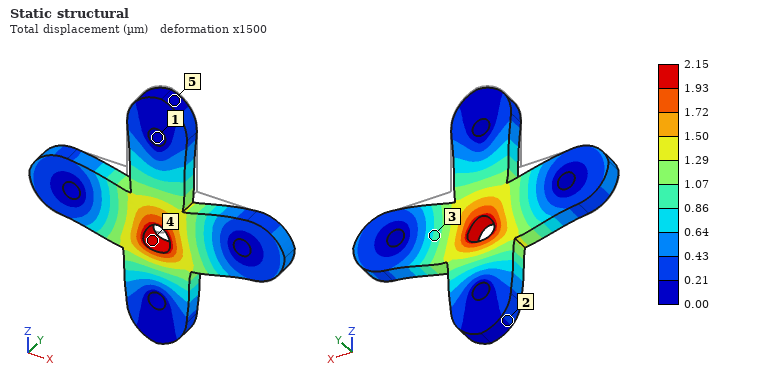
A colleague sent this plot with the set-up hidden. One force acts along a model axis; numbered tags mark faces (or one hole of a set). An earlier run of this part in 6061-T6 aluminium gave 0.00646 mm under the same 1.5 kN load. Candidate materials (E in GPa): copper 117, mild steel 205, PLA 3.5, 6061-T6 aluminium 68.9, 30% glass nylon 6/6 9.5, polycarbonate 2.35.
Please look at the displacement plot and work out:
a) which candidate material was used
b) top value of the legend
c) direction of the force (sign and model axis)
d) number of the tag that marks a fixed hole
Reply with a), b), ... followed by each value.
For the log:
a) mild steel
b) 2.15 µm
c) -Z
d) 1
